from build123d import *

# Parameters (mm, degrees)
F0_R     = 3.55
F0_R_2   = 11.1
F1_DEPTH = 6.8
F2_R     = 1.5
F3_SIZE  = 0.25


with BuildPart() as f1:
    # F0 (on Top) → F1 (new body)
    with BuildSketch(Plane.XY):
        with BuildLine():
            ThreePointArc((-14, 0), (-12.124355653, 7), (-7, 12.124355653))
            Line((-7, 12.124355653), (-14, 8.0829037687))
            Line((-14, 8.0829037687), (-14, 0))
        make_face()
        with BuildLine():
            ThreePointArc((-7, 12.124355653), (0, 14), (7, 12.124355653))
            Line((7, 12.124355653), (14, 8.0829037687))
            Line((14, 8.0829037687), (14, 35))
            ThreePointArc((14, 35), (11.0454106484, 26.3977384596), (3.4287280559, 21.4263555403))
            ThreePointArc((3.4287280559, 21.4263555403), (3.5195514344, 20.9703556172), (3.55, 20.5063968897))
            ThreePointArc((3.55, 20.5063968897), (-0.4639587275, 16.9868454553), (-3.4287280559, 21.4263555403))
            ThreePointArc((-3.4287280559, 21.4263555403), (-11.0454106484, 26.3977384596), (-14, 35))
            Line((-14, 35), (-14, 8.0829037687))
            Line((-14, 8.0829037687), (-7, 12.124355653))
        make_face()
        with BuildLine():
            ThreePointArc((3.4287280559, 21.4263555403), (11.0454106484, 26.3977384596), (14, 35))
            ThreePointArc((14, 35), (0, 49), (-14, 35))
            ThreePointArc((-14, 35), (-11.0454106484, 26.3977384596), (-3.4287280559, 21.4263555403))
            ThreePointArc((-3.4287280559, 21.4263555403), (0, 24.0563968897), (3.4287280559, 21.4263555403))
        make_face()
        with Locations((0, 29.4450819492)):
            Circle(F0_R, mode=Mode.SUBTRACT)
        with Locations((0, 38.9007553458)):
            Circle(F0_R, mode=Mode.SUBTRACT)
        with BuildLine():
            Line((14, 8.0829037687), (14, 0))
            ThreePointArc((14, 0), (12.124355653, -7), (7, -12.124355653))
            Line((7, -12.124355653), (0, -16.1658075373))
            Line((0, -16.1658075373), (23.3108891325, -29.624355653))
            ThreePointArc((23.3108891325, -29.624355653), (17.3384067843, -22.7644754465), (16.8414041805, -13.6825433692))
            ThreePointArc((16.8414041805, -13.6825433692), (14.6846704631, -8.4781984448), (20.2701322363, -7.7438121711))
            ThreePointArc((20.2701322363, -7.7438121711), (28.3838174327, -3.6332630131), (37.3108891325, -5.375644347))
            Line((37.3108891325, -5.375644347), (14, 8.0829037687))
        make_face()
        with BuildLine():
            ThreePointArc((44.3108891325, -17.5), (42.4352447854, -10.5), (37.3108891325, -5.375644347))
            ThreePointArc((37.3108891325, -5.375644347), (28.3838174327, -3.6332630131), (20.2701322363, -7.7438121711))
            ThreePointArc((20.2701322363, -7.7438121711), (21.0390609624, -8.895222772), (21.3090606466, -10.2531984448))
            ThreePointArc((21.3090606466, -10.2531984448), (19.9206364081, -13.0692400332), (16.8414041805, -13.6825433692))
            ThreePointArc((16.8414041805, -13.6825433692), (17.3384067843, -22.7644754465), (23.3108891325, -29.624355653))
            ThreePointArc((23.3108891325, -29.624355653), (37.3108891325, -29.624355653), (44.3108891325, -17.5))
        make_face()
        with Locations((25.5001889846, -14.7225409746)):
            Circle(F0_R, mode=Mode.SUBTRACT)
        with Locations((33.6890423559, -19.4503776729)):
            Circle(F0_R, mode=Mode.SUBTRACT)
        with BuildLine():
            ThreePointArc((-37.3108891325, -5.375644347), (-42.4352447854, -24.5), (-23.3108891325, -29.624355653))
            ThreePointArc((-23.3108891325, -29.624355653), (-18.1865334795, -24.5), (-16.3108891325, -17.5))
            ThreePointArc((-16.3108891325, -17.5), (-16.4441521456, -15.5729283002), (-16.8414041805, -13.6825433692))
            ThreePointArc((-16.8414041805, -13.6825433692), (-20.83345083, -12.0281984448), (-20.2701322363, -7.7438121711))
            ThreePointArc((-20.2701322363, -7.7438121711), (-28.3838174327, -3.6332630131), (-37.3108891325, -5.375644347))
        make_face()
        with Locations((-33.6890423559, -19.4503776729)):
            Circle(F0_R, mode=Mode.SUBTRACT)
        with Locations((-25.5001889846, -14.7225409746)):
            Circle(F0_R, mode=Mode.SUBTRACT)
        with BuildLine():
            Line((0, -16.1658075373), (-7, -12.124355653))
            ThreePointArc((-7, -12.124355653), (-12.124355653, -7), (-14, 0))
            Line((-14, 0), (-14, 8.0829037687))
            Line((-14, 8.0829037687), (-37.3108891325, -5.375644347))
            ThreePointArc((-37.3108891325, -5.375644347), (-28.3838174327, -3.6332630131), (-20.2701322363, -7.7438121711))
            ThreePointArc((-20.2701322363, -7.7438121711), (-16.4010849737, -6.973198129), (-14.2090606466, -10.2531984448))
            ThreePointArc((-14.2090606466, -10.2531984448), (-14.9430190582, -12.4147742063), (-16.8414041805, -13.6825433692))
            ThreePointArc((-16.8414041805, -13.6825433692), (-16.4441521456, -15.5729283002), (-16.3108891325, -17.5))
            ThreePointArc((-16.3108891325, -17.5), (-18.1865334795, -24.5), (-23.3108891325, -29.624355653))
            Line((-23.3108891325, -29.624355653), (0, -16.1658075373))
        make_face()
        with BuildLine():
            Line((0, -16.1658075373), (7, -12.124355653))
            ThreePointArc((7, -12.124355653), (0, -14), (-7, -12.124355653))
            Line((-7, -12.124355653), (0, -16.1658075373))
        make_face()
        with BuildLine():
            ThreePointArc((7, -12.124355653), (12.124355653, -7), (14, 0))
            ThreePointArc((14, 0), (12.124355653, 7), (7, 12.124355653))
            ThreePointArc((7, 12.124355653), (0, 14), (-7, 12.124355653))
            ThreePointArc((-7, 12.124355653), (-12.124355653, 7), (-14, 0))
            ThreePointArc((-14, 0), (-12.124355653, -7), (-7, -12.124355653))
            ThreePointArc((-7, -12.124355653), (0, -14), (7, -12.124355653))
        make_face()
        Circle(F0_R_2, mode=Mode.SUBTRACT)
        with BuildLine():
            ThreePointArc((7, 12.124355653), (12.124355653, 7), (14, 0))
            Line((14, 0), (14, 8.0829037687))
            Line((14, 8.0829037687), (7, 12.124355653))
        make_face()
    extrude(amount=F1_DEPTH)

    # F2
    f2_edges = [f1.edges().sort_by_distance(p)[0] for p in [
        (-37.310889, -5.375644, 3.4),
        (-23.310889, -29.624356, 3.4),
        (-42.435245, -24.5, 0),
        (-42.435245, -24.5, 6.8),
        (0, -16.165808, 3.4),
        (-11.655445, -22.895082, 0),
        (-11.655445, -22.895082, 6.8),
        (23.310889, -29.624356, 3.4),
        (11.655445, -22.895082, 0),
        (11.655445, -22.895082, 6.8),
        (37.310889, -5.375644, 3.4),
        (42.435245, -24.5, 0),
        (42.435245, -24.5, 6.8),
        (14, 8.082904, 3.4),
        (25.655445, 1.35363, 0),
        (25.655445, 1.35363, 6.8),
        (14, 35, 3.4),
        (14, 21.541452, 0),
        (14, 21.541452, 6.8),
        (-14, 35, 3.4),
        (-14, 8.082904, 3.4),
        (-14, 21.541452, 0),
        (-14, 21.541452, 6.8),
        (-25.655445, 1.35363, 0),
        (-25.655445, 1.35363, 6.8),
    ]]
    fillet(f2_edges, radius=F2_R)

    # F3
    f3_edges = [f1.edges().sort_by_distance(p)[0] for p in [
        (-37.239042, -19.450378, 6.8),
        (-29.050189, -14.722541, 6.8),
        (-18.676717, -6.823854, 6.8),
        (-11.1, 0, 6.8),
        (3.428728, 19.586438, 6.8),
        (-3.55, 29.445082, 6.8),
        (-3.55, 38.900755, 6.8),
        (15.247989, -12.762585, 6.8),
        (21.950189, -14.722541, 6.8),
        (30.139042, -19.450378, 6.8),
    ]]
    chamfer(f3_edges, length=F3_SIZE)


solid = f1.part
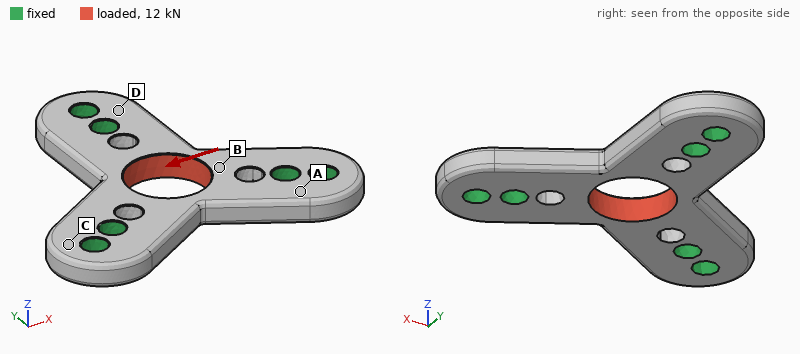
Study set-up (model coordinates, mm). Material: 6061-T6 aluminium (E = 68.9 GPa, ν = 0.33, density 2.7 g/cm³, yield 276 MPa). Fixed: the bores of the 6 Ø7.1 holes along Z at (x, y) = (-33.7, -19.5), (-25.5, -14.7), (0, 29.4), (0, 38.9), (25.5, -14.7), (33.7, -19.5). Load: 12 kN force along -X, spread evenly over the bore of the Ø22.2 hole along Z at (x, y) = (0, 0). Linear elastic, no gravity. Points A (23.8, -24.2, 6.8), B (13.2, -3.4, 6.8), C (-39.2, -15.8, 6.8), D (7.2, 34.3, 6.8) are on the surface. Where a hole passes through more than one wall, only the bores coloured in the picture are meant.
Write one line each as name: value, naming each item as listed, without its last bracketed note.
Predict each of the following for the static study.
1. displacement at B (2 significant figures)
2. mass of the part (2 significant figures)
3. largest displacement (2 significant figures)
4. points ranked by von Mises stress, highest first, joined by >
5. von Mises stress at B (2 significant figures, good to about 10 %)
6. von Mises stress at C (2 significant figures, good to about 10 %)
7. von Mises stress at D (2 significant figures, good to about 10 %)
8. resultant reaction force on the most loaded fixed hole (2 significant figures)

displacement at B: 18 µm
mass of the part: 50 g
largest displacement: 36 µm
points ranked by von Mises stress, highest first, joined by >: B > D > C > A
von Mises stress at B: 44 MPa
von Mises stress at C: 17 MPa
von Mises stress at D: 31 MPa
resultant reaction force on the most loaded fixed hole: 4.3 kN
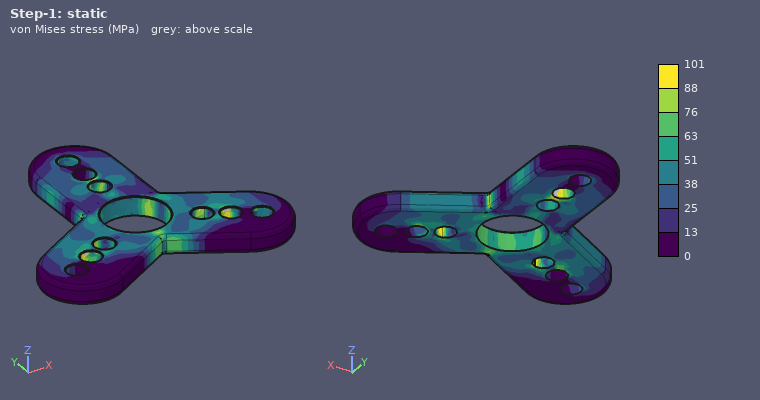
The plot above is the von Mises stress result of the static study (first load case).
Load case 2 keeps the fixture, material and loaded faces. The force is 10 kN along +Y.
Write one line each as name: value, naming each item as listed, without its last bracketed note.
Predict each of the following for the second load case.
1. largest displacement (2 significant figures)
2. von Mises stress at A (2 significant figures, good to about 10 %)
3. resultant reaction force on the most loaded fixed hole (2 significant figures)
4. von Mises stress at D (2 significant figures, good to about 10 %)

largest displacement: 33 µm
von Mises stress at A: 32 MPa
resultant reaction force on the most loaded fixed hole: 3.5 kN
von Mises stress at D: 21 MPa
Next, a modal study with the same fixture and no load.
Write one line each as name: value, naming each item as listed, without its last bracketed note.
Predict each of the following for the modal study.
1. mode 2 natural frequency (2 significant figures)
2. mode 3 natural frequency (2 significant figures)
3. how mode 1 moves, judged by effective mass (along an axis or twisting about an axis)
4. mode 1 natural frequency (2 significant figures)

mode 2 natural frequency: 17 kHz
mode 3 natural frequency: 17 kHz
how mode 1 moves, judged by effective mass: along Z
mode 1 natural frequency: 13 kHz
